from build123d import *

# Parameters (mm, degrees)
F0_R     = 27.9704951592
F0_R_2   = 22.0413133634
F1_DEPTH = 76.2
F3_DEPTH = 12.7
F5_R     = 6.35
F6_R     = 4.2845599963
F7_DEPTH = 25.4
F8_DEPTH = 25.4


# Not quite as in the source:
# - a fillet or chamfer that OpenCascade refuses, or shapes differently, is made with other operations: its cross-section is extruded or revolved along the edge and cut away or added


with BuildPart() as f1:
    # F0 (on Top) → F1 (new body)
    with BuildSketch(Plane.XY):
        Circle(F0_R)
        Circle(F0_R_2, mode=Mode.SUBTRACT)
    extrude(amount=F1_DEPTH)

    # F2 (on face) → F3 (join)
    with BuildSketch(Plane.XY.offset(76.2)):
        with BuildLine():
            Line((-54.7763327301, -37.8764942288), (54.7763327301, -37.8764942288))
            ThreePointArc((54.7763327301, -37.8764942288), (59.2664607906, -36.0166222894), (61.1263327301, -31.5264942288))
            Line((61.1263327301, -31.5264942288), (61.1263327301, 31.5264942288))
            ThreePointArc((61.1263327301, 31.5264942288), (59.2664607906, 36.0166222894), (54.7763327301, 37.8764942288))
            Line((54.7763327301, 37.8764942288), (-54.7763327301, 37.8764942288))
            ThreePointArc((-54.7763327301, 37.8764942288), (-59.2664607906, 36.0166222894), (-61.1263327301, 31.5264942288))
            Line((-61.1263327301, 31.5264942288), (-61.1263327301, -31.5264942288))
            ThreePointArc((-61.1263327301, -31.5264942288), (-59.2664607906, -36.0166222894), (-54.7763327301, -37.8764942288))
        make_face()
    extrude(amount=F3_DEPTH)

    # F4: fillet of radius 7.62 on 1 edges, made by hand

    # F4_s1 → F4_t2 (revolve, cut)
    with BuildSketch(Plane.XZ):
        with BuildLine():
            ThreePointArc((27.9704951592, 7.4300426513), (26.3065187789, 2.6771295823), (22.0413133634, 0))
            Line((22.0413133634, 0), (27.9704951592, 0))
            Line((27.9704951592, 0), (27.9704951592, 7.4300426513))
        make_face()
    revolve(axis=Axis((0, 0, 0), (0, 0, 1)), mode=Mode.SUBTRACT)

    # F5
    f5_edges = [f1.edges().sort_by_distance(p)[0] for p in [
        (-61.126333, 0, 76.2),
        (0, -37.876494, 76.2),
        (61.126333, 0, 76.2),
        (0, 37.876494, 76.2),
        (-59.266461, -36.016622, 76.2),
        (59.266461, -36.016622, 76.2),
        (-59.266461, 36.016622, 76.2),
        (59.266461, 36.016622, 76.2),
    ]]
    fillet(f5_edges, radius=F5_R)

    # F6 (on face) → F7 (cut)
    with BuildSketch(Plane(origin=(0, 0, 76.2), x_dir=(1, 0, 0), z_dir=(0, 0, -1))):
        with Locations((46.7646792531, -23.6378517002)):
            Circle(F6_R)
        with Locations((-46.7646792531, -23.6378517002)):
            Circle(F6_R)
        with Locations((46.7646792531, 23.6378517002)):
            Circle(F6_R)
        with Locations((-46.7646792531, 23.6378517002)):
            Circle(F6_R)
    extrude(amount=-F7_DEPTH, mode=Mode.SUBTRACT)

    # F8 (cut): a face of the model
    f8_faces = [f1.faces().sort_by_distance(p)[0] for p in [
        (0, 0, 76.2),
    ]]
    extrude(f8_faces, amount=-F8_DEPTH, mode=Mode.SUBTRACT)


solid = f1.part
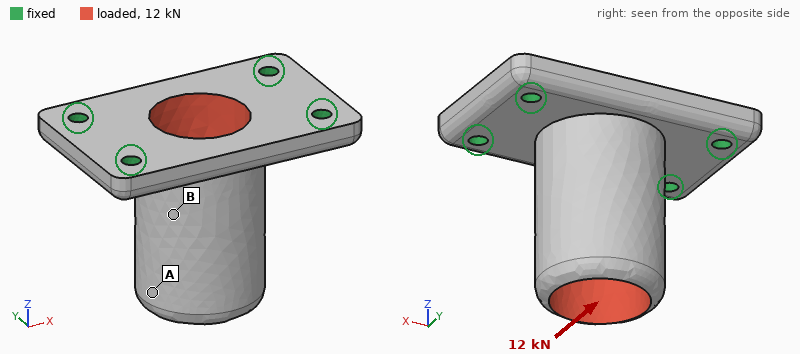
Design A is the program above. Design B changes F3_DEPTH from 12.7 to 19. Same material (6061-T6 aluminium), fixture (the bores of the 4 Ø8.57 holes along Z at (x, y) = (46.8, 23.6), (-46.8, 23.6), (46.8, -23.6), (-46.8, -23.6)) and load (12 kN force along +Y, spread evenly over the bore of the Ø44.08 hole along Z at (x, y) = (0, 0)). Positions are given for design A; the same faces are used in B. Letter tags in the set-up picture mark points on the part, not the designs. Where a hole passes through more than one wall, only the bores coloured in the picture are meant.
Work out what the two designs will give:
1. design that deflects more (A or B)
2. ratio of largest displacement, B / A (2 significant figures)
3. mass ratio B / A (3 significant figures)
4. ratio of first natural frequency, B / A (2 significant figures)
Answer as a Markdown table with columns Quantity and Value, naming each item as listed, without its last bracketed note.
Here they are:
| Quantity | Value |
|---|---|
| design that deflects more | A |
| ratio of largest displacement, B / A | 0.56 |
| mass ratio B / A | 1.29 |
| ratio of first natural frequency, B / A | 1.3 |
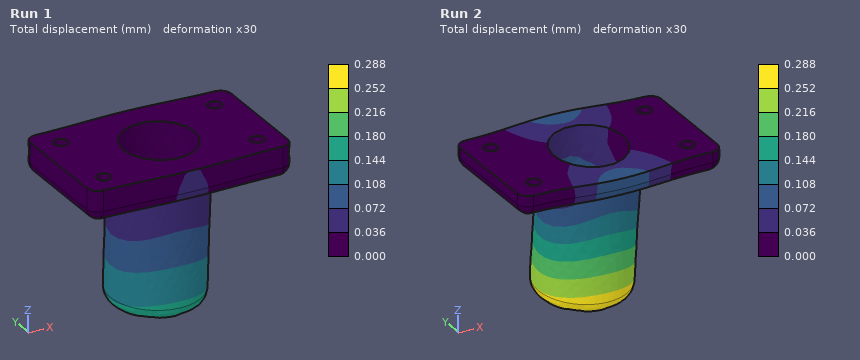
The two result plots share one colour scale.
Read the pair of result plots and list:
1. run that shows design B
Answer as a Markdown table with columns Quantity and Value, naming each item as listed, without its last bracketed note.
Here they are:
| Quantity | Value |
|---|---|
| run that shows design B | Run 1 |
